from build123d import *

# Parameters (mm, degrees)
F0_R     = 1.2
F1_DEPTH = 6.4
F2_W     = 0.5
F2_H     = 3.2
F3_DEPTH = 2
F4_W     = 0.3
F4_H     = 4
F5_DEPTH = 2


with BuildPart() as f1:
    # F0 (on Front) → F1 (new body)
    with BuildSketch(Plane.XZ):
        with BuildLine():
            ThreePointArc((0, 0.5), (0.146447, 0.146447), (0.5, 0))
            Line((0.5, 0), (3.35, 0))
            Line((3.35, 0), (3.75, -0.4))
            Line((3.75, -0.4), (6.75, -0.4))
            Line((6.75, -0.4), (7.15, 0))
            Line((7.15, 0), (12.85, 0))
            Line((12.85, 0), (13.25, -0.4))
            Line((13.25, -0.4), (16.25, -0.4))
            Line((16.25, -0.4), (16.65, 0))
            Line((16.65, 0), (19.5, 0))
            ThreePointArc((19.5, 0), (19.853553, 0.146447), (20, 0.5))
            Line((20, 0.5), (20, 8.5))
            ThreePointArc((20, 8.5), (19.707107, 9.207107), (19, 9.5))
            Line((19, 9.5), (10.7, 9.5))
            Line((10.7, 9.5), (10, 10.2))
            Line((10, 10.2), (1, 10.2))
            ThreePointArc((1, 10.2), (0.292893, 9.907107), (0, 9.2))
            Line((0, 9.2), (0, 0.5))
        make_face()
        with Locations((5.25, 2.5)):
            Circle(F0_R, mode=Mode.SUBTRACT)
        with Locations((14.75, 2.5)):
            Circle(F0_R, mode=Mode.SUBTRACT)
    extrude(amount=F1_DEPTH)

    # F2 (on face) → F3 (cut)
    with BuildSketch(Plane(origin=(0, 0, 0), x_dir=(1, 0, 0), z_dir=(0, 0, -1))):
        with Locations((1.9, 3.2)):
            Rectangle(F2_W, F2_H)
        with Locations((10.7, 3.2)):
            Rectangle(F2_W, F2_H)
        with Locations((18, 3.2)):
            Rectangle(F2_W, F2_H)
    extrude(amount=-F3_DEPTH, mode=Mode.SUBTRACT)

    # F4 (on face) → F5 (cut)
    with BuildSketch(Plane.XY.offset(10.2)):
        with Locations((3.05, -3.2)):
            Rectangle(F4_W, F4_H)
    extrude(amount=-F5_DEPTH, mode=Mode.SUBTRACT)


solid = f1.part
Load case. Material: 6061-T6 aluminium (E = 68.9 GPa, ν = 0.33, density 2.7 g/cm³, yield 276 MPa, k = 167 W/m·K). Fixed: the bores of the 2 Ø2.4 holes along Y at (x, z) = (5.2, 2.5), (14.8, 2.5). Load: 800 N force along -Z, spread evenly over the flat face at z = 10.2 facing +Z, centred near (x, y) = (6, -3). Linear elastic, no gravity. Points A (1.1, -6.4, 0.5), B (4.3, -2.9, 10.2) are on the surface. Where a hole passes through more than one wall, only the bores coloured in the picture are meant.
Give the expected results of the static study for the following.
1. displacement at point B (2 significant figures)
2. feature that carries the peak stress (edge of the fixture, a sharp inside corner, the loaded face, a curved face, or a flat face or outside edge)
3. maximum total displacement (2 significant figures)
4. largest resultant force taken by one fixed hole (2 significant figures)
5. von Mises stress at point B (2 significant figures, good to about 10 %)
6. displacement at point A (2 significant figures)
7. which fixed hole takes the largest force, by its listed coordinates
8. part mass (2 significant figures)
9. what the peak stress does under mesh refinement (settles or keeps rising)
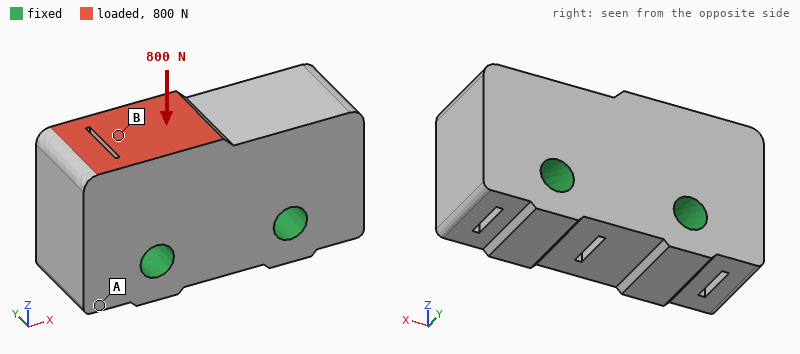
2.0 µm
edge of the fixture
2.3 µm
730 N
15 MPa
1.2 µm
(5.2, 2.5)
3.3 g
keeps rising
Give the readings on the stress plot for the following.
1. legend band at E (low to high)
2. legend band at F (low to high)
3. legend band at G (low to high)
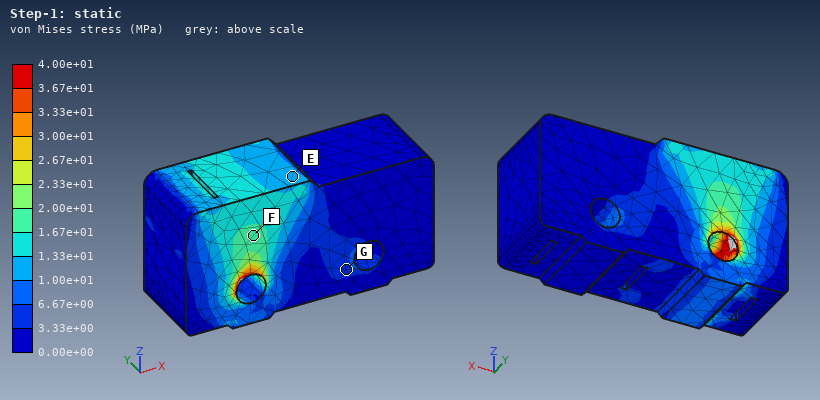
1.00e+01 to 1.33e+01 MPa
1.67e+01 to 2.00e+01 MPa
3.33e+00 to 6.67e+00 MPa
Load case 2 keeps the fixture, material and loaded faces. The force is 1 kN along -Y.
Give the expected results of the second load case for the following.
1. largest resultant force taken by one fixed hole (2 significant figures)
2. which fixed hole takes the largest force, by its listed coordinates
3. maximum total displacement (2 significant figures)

810 N
(5.2, 2.5)
17 µm
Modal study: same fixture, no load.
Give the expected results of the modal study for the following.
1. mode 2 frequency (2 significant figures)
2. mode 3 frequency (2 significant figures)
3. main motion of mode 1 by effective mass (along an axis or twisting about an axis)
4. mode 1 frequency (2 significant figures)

69 kHz
72 kHz
along Y
60 kHz
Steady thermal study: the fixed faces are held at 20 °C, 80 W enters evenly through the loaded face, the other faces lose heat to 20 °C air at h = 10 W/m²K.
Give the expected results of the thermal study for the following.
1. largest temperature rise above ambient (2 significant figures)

52 K
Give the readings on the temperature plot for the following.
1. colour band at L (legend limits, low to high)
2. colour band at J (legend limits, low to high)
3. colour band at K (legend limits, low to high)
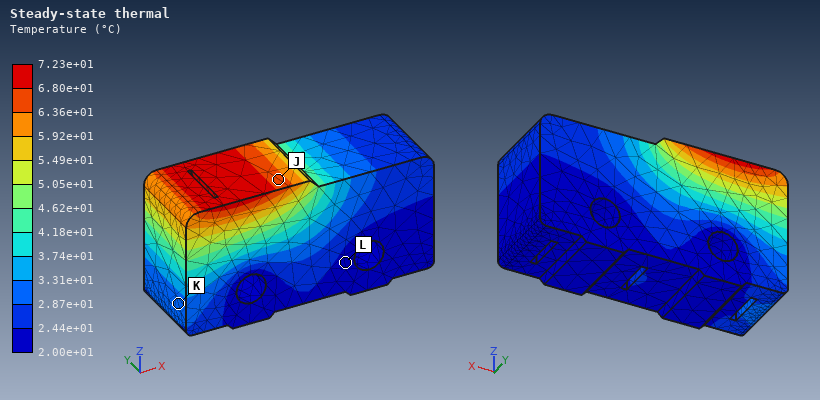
2.00e+01 to 2.44e+01 °C
6.36e+01 to 6.80e+01 °C
2.87e+01 to 3.31e+01 °C
